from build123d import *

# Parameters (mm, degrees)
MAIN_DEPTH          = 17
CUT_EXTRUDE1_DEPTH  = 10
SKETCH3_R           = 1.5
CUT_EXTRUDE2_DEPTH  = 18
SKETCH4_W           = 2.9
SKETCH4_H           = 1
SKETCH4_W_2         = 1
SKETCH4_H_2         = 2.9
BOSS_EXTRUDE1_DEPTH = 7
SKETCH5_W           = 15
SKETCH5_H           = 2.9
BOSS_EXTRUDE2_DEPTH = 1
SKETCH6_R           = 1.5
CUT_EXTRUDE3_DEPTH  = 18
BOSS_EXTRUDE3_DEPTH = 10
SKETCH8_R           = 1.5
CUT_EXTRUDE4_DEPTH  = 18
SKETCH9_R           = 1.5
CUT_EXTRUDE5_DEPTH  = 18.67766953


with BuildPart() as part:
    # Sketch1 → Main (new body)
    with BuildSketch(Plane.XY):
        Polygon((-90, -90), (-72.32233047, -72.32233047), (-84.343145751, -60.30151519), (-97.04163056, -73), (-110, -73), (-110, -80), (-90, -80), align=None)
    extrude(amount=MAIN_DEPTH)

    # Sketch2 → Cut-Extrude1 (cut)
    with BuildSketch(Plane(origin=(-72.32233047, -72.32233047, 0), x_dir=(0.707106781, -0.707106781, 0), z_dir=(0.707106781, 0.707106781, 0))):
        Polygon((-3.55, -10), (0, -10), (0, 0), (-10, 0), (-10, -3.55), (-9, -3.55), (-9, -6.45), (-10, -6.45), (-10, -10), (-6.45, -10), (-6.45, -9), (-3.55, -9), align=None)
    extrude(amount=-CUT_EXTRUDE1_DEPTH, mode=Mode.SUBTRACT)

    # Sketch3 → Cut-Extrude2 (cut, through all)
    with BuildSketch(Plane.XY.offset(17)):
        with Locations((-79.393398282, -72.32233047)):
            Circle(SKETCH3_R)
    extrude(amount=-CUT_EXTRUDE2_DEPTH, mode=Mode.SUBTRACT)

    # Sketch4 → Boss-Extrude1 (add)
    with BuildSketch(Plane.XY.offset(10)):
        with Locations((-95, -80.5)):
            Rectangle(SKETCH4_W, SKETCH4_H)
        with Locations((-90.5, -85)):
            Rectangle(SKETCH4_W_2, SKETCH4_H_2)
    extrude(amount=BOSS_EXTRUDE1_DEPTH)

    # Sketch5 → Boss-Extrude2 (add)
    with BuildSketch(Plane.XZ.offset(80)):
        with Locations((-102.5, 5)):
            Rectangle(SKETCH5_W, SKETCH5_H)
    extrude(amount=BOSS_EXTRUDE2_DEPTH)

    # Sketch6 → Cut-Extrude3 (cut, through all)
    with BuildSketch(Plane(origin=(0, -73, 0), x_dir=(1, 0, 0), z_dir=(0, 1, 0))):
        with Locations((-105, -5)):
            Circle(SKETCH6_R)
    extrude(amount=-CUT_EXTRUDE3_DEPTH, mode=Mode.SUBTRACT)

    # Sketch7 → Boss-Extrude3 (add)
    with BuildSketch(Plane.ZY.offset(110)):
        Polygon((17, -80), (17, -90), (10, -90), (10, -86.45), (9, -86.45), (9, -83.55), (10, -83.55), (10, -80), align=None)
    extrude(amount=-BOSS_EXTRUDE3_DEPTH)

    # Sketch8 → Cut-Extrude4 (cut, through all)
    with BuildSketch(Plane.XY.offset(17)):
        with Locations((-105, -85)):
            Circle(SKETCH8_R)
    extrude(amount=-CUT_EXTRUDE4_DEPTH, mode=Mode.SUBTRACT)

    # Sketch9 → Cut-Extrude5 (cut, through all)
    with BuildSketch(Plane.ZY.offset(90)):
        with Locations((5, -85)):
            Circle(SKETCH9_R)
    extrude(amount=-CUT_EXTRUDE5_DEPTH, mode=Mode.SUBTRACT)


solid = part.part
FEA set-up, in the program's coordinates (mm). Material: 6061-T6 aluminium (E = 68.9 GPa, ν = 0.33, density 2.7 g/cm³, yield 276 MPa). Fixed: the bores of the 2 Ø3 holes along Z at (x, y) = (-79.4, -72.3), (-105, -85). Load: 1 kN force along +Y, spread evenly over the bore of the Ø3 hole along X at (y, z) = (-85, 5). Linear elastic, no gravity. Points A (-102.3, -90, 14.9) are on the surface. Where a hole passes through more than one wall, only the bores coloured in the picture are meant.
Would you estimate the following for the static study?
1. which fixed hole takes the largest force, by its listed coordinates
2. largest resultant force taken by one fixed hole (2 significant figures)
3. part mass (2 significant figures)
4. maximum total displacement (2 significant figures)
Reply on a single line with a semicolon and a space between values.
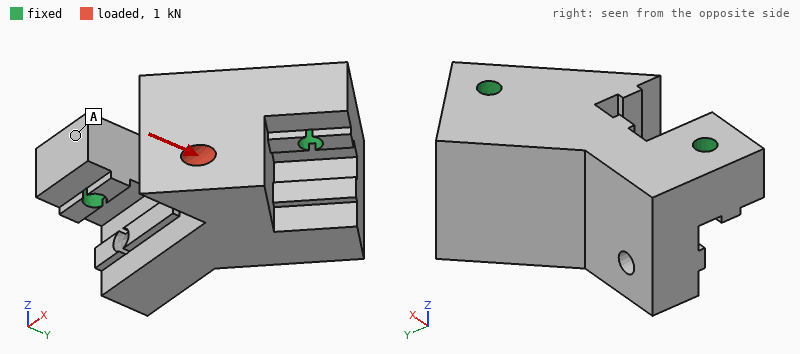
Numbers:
(-79.4, -72.3); 670 N; 20 g; 26 µm
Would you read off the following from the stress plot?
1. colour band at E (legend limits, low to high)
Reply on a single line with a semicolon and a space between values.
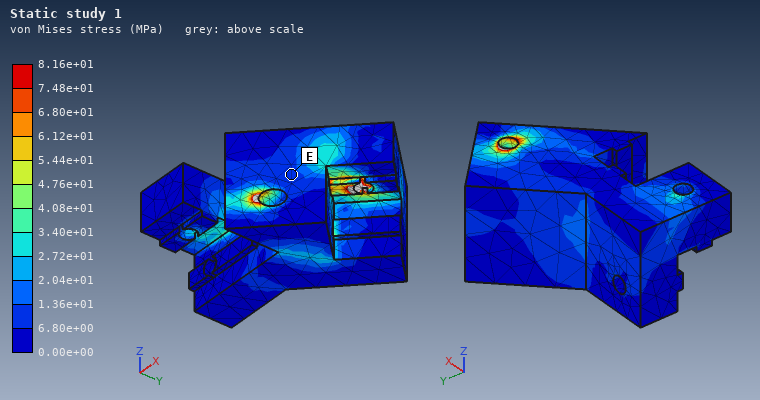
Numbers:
6.80e+00 to 1.36e+01 MPa
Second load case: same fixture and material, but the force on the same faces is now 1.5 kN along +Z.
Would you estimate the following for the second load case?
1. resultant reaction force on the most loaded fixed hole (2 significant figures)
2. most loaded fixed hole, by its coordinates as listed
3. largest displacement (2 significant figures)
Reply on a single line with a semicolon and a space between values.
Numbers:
1.0 kN; (-79.4, -72.3); 54 µm
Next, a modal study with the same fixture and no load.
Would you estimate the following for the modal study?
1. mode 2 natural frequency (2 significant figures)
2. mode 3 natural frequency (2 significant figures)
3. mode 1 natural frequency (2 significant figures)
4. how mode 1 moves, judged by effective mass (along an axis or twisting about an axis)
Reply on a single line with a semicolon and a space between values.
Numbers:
20 kHz; 25 kHz; 12 kHz; along Y
